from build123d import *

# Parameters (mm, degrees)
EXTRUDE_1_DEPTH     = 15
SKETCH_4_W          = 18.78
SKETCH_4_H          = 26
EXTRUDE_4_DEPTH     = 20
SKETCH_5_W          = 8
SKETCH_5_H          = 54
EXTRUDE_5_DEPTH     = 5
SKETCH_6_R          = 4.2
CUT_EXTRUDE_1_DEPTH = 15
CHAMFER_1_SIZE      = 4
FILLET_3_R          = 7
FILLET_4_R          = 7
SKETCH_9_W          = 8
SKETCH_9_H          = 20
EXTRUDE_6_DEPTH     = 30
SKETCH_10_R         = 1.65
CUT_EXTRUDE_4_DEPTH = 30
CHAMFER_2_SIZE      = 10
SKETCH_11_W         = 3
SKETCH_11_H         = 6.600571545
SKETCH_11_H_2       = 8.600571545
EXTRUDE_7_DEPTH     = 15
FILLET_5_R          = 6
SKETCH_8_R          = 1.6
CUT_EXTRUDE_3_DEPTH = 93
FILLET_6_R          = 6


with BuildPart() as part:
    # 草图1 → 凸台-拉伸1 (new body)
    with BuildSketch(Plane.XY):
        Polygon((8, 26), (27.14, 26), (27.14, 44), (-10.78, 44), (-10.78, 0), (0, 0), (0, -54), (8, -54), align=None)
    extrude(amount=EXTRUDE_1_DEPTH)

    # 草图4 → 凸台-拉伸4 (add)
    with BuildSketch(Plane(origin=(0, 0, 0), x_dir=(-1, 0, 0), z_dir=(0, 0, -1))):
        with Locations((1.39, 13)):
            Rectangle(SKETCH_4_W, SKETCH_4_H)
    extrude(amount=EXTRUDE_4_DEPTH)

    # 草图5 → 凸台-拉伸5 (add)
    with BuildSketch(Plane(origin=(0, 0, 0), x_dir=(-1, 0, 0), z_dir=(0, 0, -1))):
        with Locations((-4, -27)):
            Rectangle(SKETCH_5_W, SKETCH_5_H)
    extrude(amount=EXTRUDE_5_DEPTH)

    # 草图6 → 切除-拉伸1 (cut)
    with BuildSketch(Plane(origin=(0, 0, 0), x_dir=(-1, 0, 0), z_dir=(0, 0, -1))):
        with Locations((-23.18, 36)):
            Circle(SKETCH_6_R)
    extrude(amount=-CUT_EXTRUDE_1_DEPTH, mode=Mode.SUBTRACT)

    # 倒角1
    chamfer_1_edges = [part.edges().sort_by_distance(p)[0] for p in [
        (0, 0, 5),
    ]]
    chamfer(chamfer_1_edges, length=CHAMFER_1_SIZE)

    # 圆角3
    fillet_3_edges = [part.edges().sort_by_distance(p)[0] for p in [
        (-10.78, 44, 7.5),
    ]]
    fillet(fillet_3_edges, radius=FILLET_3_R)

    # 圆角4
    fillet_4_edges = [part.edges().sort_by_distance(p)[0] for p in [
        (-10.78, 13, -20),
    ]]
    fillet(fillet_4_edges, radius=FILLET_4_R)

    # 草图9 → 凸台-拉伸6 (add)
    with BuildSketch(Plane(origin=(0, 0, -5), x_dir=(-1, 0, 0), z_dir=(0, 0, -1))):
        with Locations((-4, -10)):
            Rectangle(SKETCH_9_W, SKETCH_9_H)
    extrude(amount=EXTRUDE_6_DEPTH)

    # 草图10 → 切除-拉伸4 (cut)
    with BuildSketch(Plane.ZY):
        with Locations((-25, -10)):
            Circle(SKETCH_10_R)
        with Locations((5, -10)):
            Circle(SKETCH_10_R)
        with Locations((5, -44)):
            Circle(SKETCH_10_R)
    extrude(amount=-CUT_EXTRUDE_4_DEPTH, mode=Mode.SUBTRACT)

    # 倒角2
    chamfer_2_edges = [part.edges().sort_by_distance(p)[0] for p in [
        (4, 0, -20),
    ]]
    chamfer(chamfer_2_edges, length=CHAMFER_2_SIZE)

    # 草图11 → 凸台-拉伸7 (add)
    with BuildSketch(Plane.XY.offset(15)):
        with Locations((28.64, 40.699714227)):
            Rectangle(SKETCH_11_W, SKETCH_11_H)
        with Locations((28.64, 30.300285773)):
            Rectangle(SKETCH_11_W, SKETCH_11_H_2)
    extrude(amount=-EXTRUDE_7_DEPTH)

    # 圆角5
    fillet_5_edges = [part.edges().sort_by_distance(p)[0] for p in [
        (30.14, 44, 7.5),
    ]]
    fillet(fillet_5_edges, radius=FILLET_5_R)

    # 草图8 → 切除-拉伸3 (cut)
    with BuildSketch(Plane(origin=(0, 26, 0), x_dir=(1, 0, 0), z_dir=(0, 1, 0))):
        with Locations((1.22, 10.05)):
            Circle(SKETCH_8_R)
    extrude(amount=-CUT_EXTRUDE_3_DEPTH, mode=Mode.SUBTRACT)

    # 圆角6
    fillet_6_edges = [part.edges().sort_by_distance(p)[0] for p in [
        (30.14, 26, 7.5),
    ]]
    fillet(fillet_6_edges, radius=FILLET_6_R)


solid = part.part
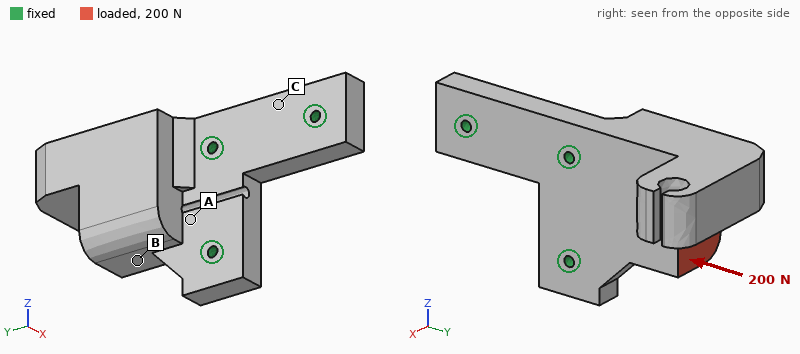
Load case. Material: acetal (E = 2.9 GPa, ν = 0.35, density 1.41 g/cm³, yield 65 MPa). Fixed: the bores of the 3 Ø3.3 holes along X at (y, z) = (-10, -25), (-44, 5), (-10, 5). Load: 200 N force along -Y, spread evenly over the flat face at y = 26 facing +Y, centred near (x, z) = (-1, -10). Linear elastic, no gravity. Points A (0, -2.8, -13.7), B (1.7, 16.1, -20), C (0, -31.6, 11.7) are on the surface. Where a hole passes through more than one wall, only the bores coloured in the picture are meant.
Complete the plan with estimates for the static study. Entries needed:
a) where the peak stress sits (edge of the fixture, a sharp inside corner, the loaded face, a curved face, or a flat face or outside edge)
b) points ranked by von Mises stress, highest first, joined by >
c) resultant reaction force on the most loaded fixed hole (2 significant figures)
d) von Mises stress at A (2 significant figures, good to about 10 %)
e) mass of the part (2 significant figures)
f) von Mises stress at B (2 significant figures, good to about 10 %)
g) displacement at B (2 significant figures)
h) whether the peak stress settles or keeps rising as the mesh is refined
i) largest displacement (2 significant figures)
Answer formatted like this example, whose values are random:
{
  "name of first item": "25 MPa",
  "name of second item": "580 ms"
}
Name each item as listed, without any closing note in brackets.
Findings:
{
  "where the peak stress sits": "edge of the fixture",
  "points ranked by von Mises stress, highest first, joined by >": "A > B > C",
  "resultant reaction force on the most loaded fixed hole": "97 N",
  "von Mises stress at A": "2.3 MPa",
  "mass of the part": "56 g",
  "von Mises stress at B": "0.81 MPa",
  "displacement at B": "0.060 mm",
  "whether the peak stress settles or keeps rising as the mesh is refined": "keeps rising",
  "largest displacement": "0.15 mm"
}
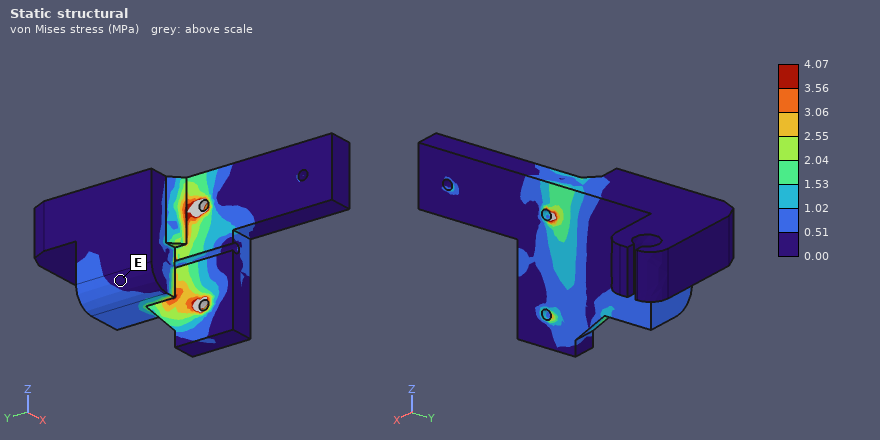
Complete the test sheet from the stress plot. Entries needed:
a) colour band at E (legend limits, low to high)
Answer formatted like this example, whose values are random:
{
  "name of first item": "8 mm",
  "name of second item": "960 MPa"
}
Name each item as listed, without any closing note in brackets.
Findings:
{
  "colour band at E": "0.00 to 0.51 MPa"
}
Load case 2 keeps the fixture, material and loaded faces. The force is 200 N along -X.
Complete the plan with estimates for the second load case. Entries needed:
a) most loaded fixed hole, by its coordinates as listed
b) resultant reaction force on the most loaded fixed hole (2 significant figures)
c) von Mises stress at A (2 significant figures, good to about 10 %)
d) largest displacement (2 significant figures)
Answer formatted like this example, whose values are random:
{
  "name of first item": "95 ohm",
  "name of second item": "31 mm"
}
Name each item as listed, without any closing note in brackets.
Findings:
{
  "most loaded fixed hole, by its coordinates as listed": "(-10, 5)",
  "resultant reaction force on the most loaded fixed hole": "140 N",
  "von Mises stress at A": "9.1 MPa",
  "largest displacement": "0.95 mm"
}
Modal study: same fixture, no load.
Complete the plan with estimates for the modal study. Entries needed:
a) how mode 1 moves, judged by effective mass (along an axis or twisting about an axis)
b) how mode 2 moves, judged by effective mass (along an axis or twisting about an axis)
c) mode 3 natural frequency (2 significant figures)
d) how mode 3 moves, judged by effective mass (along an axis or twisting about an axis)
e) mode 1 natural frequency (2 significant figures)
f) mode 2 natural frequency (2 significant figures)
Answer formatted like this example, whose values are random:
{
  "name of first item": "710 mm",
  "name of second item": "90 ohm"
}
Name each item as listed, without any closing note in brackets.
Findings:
{
  "how mode 1 moves, judged by effective mass": "along X",
  "how mode 2 moves, judged by effective mass": "along Z",
  "mode 3 natural frequency": "2200 Hz",
  "how mode 3 moves, judged by effective mass": "along Z",
  "mode 1 natural frequency": "490 Hz",
  "mode 2 natural frequency": "1500 Hz"
}
